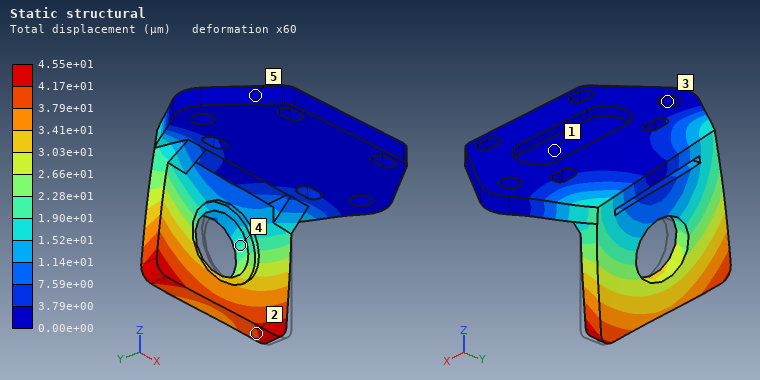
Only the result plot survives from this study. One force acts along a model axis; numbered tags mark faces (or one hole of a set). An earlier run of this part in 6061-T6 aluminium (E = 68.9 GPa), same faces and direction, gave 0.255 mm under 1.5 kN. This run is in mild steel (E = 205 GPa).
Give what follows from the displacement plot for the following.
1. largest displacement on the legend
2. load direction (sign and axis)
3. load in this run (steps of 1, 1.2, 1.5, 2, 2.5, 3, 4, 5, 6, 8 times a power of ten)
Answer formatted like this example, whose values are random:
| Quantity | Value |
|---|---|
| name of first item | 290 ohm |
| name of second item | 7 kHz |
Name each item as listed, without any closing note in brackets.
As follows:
| Quantity | Value |
|---|---|
| largest displacement on the legend | 4.55e+01 µm |
| load direction | -X |
| load in this run | 800 N |
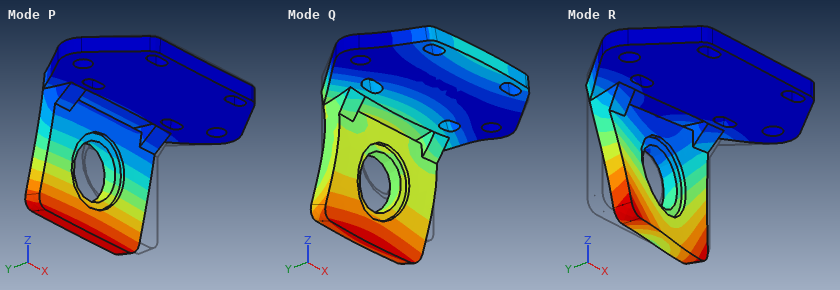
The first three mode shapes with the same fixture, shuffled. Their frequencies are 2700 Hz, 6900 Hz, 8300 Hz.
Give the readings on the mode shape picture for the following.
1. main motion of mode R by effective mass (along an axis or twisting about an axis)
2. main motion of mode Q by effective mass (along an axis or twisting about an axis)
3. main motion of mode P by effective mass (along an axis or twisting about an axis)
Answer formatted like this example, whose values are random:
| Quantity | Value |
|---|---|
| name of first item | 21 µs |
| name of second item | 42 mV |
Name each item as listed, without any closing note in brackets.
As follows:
| Quantity | Value |
|---|---|
| main motion of mode R by effective mass | along X |
| main motion of mode Q by effective mass | along Z |
| main motion of mode P by effective mass | along Y |
